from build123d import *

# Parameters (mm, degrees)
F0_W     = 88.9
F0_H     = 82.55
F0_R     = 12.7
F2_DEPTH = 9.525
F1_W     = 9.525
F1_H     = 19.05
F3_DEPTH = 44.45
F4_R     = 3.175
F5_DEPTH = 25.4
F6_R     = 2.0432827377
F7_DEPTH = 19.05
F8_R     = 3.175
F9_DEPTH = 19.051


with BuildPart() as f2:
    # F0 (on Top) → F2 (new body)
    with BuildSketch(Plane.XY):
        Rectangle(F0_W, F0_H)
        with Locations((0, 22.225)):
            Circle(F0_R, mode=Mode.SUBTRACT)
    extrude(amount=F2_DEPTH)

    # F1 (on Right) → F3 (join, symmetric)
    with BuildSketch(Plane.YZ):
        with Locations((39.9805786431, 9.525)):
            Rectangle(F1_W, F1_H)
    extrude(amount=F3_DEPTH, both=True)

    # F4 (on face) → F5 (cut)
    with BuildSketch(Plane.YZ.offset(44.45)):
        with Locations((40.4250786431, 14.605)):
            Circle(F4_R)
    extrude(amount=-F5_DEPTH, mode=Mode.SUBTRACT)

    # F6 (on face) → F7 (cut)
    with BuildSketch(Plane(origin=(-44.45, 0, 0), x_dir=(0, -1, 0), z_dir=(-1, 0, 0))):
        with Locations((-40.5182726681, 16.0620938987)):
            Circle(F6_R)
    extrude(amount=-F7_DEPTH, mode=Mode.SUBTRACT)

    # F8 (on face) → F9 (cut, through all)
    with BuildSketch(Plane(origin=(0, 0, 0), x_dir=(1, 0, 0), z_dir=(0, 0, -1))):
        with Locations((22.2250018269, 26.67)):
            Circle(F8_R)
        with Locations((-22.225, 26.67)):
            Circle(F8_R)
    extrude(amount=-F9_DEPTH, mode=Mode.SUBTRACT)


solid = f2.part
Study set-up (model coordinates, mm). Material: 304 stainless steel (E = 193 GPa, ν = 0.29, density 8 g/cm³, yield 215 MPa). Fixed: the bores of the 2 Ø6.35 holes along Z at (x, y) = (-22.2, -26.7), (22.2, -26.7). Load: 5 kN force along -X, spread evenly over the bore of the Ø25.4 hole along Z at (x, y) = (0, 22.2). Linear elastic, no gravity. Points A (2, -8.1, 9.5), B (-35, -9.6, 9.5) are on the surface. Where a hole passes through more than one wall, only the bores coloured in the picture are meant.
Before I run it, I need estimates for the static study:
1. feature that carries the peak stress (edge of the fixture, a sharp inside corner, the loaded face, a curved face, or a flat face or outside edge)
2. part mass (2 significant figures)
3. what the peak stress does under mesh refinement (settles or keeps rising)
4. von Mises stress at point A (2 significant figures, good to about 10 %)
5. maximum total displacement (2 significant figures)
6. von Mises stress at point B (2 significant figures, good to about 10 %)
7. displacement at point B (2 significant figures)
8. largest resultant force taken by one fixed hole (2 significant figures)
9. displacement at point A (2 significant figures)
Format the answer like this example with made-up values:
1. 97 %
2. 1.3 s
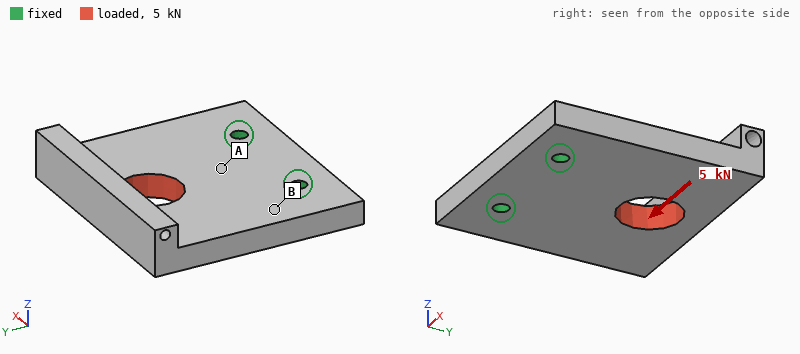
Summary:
1. edge of the fixture
2. 600 g
3. keeps rising
4. 24 MPa
5. 17 µm
6. 8.9 MPa
7. 5.2 µm
8. 5.6 kN
9. 3.6 µm
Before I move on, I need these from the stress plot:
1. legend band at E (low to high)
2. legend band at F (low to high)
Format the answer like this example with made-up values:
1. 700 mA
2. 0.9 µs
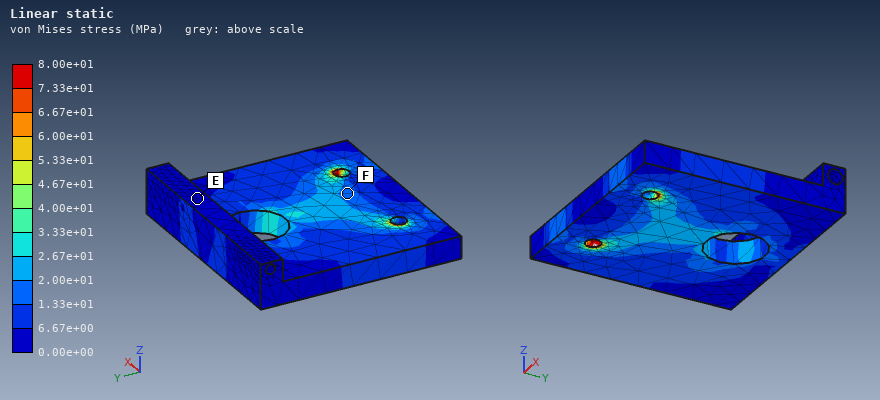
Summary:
1. 0.00e+00 to 6.67e+00 MPa
2. 1.33e+01 to 2.00e+01 MPa
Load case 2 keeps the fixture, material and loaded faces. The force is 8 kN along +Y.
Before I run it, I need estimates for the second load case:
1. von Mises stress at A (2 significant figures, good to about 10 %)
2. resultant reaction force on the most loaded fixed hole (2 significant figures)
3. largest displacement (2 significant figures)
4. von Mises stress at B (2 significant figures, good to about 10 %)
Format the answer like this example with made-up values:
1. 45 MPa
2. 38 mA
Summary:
1. 9.8 MPa
2. 4.0 kN
3. 7.6 µm
4. 6.8 MPa
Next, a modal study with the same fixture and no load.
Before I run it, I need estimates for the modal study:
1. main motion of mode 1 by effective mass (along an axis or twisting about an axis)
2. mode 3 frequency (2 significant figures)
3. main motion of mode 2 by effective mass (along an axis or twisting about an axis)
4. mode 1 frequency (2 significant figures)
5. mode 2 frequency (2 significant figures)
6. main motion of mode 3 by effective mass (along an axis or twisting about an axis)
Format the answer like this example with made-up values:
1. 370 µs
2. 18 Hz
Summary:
1. along Z
2. 5000 Hz
3. twisting about Y
4. 1200 Hz
5. 2400 Hz
6. along X
